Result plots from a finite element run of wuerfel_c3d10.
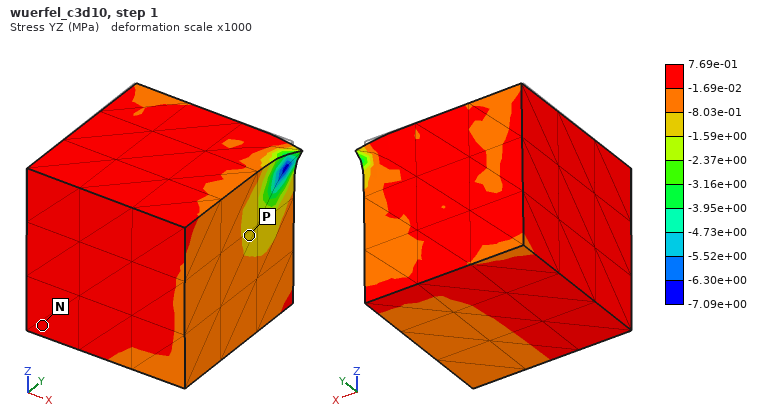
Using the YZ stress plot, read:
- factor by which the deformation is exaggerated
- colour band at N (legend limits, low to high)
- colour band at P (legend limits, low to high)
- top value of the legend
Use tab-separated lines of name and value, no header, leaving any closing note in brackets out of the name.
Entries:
factor by which the deformation is exaggerated	1000
colour band at N	-1.69e-02 to 7.69e-01 MPa
colour band at P	-1.59e+00 to -8.03e-01 MPa
top value of the legend	7.69e-01 MPa
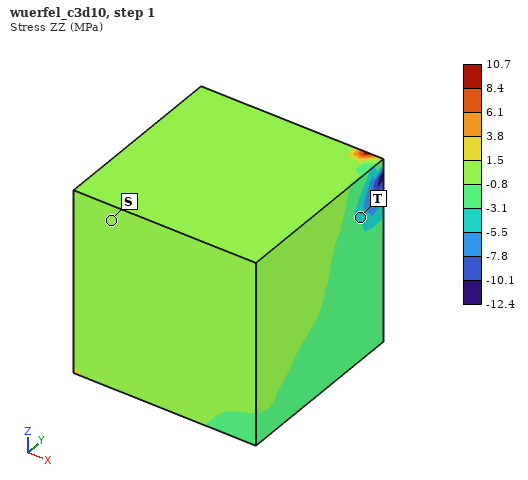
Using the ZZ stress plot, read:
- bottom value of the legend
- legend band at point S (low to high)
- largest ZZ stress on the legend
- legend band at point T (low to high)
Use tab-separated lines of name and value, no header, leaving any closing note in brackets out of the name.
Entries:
bottom value of the legend	-12.4 MPa
legend band at point S	-0.8 to 1.5 MPa
largest ZZ stress on the legend	10.7 MPa
legend band at point T	-5.5 to -3.1 MPa
